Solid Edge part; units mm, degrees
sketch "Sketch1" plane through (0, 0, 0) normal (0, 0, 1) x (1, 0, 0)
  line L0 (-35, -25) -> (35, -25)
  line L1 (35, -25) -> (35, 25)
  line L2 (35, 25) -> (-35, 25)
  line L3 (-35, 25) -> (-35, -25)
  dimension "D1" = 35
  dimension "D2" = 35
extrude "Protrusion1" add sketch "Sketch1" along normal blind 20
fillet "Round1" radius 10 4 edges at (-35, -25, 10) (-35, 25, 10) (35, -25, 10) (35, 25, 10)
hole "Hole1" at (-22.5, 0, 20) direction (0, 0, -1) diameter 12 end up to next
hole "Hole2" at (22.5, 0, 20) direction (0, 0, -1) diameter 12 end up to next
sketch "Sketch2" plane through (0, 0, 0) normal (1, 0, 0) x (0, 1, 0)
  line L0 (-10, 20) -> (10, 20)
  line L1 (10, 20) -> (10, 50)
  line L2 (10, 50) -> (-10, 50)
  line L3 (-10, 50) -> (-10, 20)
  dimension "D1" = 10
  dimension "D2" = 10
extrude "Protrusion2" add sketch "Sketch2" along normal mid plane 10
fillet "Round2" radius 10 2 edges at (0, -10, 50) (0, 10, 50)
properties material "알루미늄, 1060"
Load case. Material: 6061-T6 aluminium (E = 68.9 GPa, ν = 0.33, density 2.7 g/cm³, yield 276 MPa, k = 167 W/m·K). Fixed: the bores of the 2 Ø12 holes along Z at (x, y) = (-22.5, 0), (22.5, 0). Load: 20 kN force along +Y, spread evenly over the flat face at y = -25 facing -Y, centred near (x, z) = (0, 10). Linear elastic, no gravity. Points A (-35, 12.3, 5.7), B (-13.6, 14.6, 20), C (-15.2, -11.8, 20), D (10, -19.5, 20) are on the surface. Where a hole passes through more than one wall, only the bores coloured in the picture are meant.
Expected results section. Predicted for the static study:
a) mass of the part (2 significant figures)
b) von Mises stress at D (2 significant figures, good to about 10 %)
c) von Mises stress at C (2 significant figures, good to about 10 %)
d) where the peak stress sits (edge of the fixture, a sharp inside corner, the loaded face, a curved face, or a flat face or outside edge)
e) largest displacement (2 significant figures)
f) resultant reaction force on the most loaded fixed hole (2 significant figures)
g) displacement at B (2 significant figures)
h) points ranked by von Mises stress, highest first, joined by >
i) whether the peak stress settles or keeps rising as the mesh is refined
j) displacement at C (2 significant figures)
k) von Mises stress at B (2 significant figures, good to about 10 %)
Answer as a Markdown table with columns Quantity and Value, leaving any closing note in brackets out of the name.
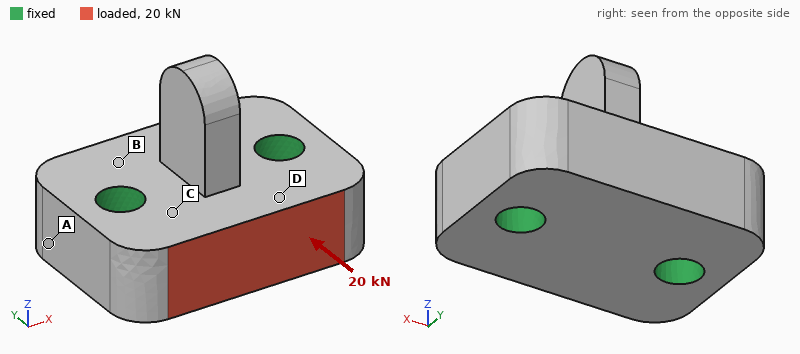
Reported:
| Quantity | Value |
|---|---|
| mass of the part | 190 g |
| von Mises stress at D | 18 MPa |
| von Mises stress at C | 23 MPa |
| where the peak stress sits | edge of the fixture |
| largest displacement | 9.3 µm |
| resultant reaction force on the most loaded fixed hole | 10 kN |
| displacement at B | 1.8 µm |
| points ranked by von Mises stress, highest first, joined by > | C > D > B > A |
| whether the peak stress settles or keeps rising as the mesh is refined | keeps rising |
| displacement at C | 3.6 µm |
| von Mises stress at B | 7.1 MPa |
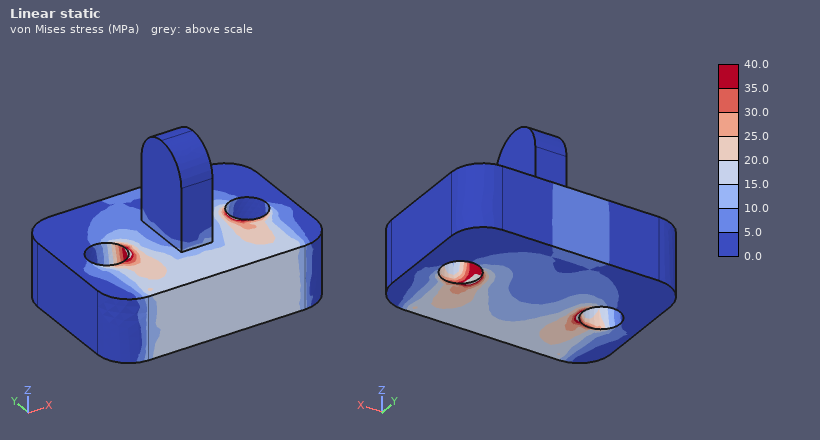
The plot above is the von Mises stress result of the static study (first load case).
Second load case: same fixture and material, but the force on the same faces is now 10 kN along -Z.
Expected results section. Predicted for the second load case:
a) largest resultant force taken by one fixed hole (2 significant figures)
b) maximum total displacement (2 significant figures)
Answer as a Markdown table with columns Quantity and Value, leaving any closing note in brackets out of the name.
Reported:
| Quantity | Value |
|---|---|
| largest resultant force taken by one fixed hole | 5.0 kN |
| maximum total displacement | 33 µm |
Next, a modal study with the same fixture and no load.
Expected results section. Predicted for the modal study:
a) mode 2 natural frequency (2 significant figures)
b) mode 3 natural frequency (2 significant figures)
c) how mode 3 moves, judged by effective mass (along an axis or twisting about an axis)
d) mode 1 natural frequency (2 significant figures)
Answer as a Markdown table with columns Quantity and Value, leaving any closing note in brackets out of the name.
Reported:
| Quantity | Value |
|---|---|
| mode 2 natural frequency | 11 kHz |
| mode 3 natural frequency | 20 kHz |
| how mode 3 moves, judged by effective mass | along Z |
| mode 1 natural frequency | 8100 Hz |
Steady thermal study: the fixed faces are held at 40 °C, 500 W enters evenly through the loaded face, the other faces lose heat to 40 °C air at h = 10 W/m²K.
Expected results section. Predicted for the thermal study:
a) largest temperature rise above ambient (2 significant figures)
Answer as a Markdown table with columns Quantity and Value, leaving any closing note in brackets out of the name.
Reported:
| Quantity | Value |
|---|---|
| largest temperature rise above ambient | 66 K |
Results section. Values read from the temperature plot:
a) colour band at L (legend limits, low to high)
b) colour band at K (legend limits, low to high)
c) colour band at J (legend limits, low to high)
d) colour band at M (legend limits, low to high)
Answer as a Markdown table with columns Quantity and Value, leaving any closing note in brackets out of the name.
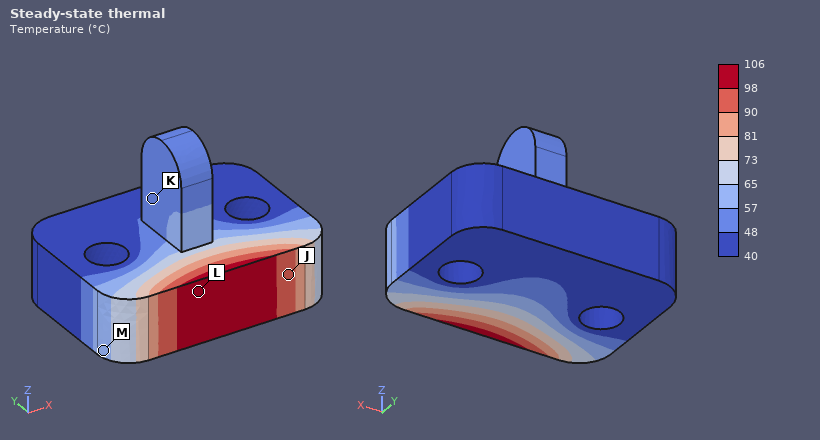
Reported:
| Quantity | Value |
|---|---|
| colour band at L | 98 to 106 °C |
| colour band at K | 48 to 57 °C |
| colour band at J | 90 to 98 °C |
| colour band at M | 57 to 65 °C |
